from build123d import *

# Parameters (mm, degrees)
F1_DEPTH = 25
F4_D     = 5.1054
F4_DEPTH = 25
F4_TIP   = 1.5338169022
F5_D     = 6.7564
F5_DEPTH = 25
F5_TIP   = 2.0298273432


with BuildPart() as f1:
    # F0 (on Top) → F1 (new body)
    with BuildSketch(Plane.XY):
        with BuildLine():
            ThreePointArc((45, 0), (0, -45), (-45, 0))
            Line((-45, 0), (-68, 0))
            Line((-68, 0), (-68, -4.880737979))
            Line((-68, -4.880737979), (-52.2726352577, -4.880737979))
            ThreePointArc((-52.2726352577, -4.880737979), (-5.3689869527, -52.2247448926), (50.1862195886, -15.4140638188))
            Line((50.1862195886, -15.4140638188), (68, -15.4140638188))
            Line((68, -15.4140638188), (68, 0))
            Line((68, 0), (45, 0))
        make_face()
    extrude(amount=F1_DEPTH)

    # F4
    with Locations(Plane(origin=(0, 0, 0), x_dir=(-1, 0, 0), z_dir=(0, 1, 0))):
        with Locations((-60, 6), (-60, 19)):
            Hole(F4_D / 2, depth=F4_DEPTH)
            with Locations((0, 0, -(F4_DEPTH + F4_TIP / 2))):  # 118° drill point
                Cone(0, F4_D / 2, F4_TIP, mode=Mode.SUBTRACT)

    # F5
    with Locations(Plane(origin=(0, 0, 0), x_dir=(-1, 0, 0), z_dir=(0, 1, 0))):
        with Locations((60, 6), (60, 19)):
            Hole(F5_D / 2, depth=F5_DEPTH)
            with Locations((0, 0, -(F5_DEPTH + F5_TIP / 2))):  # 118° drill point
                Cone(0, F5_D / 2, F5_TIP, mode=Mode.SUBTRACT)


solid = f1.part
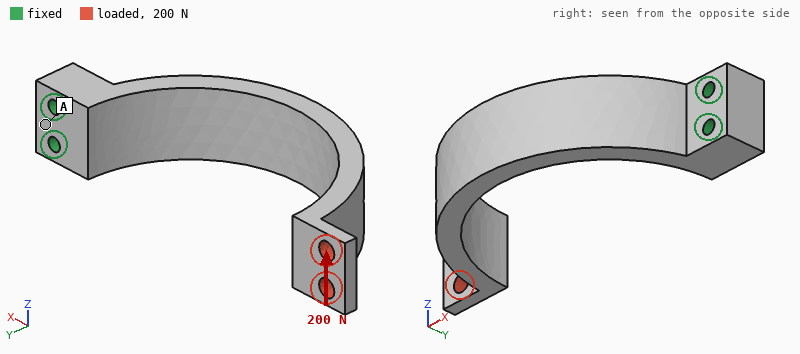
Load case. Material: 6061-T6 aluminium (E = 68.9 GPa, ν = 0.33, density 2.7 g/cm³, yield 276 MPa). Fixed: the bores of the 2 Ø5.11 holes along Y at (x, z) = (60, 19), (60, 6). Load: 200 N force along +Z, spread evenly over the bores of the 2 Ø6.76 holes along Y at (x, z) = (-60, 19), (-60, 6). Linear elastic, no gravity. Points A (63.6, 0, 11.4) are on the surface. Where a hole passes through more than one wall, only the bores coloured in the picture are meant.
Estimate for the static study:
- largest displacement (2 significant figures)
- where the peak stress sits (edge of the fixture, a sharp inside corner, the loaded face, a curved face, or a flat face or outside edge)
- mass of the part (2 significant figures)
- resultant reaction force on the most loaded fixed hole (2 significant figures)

1.4 mm
a curved face
97 g
1.5 kN
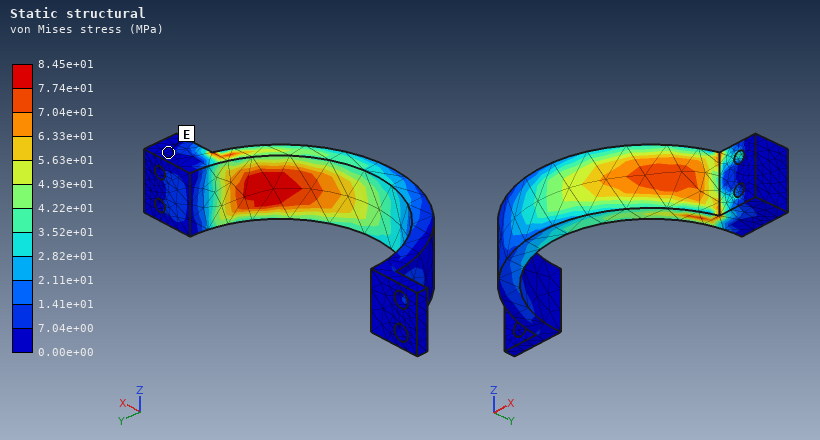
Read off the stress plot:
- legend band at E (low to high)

0.00e+00 to 7.04e+00 MPa
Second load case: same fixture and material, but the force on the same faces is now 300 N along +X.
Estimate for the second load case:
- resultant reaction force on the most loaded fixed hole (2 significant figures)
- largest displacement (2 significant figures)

150 N
1.7 mm
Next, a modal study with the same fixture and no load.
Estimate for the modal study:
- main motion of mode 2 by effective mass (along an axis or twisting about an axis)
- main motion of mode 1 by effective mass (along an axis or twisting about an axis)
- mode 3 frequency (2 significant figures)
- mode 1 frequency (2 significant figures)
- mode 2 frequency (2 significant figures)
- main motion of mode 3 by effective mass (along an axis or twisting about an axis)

along Z
along Y
1000 Hz
320 Hz
470 Hz
along X
